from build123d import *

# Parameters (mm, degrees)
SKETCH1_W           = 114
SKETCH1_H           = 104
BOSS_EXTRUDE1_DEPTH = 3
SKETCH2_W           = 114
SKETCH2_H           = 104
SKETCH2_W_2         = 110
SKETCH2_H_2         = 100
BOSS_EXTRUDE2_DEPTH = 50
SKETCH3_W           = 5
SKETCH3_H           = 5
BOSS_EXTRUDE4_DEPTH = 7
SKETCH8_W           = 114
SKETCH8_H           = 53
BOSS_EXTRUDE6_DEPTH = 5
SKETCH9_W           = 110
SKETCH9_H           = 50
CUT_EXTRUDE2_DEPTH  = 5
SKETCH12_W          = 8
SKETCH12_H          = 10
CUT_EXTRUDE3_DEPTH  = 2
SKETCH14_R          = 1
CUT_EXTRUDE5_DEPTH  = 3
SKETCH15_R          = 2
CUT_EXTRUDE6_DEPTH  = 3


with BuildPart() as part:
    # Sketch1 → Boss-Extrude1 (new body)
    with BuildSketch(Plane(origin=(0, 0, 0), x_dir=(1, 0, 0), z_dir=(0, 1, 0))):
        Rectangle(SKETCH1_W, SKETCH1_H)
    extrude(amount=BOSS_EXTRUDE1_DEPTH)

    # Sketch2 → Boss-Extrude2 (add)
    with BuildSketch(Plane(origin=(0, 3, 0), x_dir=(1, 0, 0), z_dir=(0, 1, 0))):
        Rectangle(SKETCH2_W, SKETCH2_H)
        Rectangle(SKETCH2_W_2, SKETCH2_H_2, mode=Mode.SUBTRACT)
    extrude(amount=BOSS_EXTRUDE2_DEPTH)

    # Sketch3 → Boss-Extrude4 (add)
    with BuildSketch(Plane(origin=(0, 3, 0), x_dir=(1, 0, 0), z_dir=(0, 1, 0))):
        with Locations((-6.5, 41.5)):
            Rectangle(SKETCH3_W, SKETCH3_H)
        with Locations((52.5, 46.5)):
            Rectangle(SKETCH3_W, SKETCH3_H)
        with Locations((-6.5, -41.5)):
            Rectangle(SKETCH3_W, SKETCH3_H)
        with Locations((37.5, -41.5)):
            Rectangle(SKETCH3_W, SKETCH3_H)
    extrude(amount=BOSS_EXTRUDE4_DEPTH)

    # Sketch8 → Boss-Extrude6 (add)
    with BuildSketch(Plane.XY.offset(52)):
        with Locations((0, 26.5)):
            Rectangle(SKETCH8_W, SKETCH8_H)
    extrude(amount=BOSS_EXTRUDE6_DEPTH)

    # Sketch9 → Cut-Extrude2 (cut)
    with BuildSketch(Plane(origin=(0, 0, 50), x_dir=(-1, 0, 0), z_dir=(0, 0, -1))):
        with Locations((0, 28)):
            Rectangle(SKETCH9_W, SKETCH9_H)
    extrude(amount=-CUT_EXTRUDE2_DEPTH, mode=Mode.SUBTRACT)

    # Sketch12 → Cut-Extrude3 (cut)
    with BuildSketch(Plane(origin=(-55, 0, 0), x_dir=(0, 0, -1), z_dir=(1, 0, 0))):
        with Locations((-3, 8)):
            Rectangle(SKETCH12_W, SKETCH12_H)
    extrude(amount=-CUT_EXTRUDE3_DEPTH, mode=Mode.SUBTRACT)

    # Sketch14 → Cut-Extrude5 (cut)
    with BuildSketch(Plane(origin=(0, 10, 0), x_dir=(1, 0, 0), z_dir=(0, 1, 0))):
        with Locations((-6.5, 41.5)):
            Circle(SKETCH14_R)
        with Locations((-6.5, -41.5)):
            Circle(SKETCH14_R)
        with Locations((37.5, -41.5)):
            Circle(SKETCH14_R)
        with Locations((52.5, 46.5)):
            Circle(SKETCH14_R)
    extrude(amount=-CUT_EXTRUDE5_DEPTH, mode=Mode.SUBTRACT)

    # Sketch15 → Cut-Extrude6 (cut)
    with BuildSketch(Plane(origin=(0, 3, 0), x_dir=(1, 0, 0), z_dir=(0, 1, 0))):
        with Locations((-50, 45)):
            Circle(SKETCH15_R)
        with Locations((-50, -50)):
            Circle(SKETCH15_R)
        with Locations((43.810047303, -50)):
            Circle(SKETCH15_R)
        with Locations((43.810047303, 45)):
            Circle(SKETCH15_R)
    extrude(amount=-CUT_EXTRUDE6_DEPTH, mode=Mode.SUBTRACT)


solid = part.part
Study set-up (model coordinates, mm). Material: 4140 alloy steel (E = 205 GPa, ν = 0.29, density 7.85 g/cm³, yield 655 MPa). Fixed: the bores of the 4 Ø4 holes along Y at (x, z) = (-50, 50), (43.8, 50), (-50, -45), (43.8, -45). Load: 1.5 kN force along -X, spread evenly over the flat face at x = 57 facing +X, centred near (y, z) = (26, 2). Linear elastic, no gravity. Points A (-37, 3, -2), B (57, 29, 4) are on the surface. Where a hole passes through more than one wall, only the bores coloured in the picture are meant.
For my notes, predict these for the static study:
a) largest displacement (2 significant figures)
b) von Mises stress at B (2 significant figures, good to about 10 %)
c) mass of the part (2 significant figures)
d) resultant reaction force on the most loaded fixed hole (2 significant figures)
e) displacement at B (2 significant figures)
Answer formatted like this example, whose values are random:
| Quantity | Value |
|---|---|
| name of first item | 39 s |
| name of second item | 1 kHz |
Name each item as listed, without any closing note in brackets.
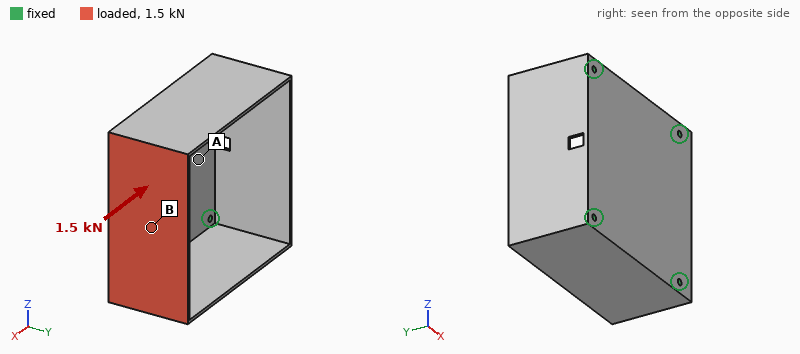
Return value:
| Quantity | Value |
|---|---|
| largest displacement | 0.62 mm |
| von Mises stress at B | 57 MPa |
| mass of the part | 640 g |
| resultant reaction force on the most loaded fixed hole | 450 N |
| displacement at B | 0.30 mm |
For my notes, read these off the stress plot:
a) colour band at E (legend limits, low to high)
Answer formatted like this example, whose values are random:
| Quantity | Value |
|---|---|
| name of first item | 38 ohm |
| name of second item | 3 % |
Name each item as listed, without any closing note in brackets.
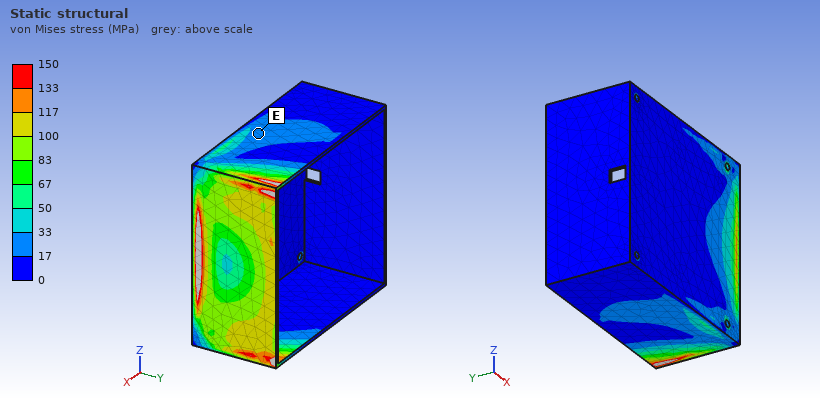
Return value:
| Quantity | Value |
|---|---|
| colour band at E | 17 to 33 MPa |
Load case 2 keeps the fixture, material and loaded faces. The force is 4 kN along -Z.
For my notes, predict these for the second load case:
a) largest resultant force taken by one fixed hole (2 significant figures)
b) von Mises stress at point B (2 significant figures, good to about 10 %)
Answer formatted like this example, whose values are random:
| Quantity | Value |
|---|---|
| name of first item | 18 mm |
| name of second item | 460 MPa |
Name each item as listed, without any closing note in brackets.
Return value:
| Quantity | Value |
|---|---|
| largest resultant force taken by one fixed hole | 2.2 kN |
| von Mises stress at point B | 16 MPa |
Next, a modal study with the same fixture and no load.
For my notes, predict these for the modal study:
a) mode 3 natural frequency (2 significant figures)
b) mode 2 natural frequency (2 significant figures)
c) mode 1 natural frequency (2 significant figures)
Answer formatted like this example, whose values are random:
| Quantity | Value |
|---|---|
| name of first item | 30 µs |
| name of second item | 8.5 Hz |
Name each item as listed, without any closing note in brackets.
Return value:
| Quantity | Value |
|---|---|
| mode 3 natural frequency | 1100 Hz |
| mode 2 natural frequency | 1100 Hz |
| mode 1 natural frequency | 960 Hz |
